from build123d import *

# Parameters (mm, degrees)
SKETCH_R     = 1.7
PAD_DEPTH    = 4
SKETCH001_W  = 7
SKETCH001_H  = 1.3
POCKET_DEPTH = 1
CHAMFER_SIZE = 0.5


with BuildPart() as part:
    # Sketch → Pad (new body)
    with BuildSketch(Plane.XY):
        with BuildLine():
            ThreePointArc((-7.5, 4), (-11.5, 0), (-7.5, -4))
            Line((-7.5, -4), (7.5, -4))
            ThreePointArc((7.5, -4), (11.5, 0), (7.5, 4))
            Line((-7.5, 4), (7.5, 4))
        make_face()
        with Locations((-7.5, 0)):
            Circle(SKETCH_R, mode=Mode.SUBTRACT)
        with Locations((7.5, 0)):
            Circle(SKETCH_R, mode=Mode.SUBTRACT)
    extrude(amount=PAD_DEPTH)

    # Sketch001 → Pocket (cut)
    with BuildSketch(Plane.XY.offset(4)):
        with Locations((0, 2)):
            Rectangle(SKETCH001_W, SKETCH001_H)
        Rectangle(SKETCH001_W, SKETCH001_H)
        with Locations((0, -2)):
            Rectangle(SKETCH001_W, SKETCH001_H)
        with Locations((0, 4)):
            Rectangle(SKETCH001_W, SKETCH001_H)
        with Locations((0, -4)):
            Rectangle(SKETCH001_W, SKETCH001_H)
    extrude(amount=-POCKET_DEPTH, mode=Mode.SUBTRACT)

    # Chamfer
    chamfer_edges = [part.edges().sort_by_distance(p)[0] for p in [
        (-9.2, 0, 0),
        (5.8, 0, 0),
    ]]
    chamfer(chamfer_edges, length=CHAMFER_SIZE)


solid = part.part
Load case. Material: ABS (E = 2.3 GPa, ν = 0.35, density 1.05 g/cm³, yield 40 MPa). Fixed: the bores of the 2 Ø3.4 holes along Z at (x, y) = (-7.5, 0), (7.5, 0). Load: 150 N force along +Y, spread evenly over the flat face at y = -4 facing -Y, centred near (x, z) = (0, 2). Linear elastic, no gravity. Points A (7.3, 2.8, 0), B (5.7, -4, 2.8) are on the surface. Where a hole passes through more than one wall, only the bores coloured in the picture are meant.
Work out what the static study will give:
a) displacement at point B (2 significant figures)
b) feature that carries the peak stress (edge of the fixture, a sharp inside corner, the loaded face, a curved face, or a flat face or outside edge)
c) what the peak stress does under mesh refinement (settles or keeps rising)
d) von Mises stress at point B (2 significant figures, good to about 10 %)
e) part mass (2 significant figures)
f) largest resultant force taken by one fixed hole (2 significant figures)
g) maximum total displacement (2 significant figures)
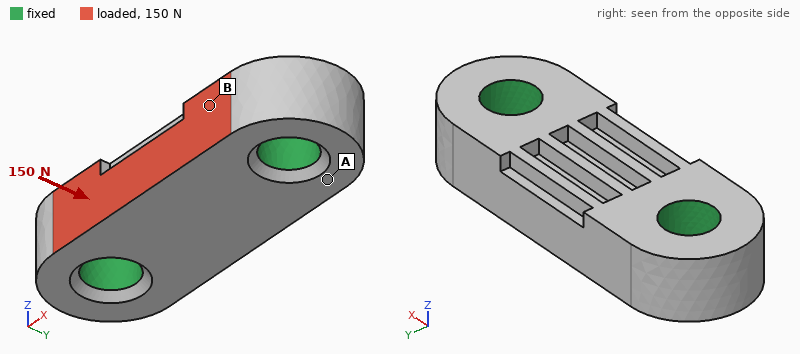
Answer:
7.8 µm
edge of the fixture
keeps rising
3.1 MPa
0.60 g
76 N
19 µm
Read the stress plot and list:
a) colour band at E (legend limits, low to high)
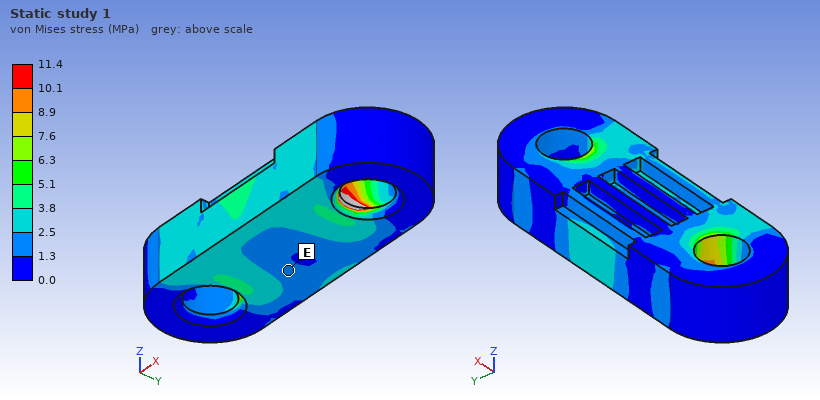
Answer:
1.3 to 2.5 MPa
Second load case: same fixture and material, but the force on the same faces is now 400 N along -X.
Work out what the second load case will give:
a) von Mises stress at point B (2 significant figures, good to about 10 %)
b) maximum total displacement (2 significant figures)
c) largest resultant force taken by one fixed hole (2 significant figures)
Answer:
14 MPa
36 µm
210 N
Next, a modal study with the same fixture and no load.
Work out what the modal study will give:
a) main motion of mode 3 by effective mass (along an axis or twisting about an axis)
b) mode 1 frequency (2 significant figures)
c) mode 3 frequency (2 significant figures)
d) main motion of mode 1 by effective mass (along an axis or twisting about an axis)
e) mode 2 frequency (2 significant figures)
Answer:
along Y
23 kHz
27 kHz
along Z
26 kHz
